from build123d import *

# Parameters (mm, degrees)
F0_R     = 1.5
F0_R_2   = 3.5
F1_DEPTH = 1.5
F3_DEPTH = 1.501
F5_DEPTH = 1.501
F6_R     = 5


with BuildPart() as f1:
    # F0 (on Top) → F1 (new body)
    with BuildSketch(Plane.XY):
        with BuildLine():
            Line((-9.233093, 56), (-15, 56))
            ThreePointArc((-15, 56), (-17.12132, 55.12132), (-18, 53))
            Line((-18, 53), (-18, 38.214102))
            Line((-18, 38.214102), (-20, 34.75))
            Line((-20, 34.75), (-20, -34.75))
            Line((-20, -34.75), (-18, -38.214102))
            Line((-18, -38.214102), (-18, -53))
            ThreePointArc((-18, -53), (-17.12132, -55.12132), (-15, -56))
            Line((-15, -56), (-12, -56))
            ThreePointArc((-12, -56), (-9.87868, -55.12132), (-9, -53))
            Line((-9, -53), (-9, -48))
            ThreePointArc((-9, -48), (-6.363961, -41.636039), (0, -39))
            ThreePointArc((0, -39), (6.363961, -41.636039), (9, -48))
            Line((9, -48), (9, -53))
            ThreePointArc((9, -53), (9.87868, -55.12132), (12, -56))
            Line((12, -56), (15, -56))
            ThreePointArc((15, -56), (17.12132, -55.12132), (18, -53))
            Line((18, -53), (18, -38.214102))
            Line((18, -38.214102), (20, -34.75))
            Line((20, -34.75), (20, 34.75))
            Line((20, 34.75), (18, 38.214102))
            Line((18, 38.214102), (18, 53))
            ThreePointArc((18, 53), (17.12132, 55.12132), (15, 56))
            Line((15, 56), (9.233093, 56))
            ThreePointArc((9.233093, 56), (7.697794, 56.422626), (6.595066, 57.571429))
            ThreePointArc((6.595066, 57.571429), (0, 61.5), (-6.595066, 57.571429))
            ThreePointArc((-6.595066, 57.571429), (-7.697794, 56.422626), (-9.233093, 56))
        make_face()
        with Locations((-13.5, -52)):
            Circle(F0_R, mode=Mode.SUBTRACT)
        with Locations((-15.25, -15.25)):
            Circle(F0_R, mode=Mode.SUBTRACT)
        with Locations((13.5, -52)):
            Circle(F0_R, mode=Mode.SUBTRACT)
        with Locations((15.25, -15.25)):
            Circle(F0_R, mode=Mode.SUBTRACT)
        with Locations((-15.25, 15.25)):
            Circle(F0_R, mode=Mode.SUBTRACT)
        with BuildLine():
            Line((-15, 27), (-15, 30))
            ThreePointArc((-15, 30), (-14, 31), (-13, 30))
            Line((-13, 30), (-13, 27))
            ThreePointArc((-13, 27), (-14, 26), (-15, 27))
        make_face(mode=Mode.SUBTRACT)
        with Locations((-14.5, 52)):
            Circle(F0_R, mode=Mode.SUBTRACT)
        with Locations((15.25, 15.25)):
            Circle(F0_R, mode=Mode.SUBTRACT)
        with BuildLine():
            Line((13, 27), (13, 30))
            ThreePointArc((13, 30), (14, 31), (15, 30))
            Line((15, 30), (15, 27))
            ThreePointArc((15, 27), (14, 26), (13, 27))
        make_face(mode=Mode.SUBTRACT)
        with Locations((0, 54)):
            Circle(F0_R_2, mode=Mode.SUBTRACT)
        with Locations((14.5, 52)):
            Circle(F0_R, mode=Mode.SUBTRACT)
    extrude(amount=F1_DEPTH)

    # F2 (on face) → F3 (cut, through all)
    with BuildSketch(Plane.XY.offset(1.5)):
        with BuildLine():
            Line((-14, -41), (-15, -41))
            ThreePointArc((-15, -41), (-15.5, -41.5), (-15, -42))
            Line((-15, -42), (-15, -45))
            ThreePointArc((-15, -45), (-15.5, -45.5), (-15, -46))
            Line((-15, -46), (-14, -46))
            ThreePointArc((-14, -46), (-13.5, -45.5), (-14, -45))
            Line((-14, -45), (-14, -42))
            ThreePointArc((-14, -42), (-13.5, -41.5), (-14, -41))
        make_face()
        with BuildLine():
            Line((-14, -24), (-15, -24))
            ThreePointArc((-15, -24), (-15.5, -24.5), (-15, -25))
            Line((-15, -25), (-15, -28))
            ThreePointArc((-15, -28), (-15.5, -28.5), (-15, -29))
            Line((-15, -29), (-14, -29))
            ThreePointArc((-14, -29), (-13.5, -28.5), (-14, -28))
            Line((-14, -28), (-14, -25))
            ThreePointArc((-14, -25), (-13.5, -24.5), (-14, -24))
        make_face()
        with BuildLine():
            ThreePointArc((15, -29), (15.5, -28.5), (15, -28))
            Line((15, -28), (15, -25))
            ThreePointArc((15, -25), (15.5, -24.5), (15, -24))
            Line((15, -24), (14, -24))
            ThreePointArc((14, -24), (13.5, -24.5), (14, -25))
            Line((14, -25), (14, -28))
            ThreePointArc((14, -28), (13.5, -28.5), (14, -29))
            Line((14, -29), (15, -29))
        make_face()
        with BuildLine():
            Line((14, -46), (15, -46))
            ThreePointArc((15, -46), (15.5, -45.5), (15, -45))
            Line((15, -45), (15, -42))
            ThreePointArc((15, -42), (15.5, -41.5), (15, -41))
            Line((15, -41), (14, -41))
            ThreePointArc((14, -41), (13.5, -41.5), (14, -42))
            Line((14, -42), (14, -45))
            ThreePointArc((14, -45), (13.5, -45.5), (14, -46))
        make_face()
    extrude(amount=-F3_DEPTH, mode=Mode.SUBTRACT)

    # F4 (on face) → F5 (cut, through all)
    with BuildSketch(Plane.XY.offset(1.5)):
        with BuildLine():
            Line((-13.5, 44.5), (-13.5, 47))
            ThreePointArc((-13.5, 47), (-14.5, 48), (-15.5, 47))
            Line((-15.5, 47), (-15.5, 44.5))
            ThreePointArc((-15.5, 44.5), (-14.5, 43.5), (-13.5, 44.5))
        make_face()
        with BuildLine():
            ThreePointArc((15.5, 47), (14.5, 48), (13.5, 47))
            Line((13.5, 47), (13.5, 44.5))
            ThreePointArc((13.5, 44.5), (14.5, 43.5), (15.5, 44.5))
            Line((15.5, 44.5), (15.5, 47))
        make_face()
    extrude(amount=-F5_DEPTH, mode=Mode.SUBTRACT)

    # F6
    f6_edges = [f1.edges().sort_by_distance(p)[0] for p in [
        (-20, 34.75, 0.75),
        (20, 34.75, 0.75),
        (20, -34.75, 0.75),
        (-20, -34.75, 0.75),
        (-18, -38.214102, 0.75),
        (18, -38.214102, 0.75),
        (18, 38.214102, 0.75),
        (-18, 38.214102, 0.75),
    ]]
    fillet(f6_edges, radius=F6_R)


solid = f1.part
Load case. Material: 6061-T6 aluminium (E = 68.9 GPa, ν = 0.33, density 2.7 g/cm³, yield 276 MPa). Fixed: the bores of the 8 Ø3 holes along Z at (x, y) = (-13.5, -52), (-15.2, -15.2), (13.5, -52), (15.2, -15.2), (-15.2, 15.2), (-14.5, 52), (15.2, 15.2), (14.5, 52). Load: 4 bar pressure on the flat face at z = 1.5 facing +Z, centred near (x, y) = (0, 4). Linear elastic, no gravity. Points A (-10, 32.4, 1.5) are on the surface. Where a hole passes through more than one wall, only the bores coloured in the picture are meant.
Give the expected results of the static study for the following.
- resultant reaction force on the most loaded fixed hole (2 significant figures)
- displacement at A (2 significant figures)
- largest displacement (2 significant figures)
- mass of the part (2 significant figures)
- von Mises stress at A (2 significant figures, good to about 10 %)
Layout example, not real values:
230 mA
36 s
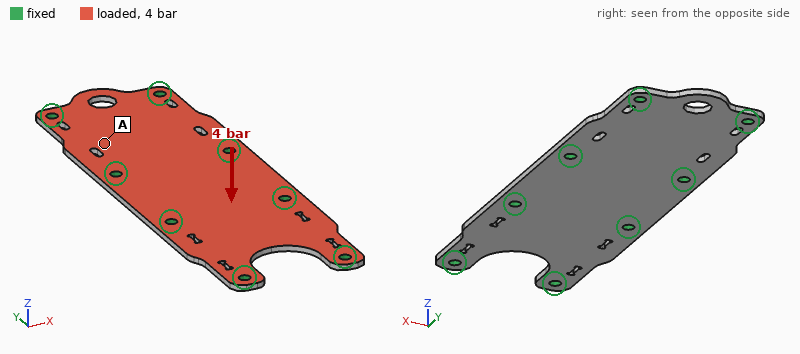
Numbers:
270 N
0.12 mm
0.14 mm
16 g
55 MPa
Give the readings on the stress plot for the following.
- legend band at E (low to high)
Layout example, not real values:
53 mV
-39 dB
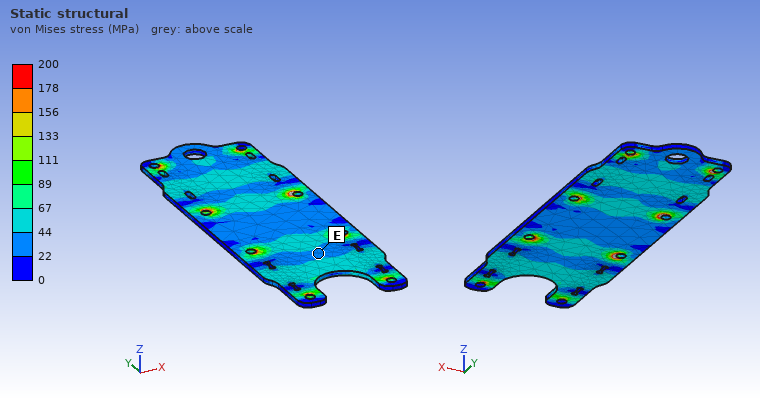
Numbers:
22 to 44 MPa
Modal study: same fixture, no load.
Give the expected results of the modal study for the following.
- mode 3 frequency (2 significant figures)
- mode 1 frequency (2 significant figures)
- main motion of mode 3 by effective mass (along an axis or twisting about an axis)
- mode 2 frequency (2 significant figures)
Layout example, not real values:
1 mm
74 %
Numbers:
6500 Hz
5000 Hz
along Z
5000 Hz
